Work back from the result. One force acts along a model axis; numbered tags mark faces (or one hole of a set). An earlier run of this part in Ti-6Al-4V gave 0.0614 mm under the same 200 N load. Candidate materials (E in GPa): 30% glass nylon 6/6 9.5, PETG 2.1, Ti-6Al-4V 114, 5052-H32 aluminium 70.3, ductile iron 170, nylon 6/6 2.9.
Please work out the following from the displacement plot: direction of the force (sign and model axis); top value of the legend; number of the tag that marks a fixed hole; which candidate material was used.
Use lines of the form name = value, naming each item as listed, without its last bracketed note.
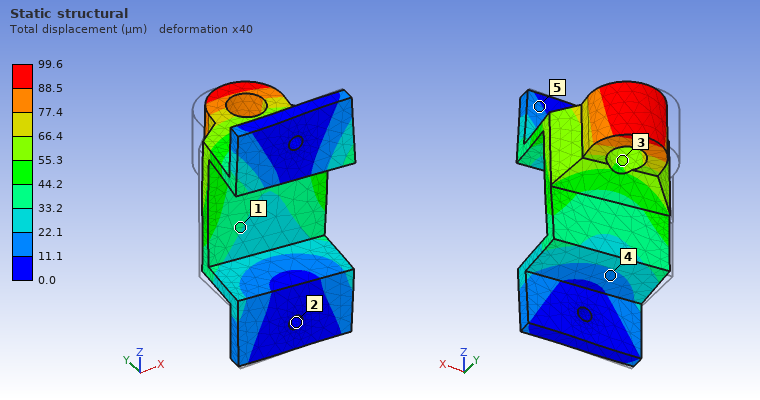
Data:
direction of the force = +X
top value of the legend = 99.6 µm
number of the tag that marks a fixed hole = 2
which candidate material was used = 5052-H32 aluminium
